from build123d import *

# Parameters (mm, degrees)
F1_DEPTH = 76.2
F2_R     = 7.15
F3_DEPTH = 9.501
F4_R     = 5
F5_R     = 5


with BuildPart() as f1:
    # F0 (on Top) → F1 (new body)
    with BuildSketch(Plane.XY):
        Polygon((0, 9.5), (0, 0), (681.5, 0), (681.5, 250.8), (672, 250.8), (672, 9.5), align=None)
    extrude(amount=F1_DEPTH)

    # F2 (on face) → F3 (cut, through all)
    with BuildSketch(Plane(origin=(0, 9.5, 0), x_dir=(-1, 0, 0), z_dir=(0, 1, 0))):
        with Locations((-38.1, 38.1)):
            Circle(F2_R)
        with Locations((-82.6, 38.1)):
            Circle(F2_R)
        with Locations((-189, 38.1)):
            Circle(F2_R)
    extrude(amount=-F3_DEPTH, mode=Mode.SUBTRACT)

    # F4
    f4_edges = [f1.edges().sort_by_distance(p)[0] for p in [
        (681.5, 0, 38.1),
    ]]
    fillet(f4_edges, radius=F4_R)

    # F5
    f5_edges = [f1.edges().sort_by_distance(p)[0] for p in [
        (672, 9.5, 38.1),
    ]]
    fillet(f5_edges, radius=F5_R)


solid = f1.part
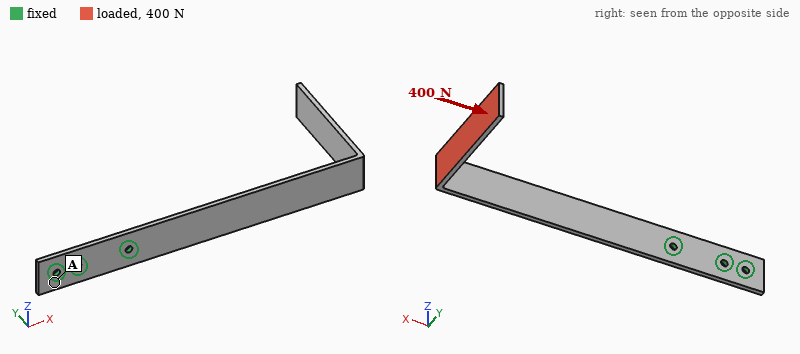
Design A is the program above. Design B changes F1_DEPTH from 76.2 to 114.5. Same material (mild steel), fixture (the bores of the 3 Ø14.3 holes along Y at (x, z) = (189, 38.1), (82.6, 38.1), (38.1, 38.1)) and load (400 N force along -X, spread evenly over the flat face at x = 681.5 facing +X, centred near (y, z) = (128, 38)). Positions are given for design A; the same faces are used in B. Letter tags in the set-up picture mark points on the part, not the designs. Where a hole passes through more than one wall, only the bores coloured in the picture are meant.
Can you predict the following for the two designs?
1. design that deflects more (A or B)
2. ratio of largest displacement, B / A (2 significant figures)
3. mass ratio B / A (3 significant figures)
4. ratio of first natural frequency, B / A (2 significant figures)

A
0.67
1.51
0.99
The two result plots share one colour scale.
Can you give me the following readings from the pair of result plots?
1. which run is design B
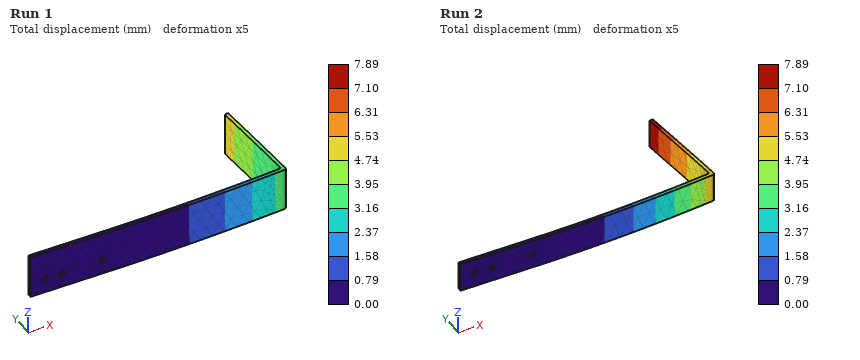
Run 1
